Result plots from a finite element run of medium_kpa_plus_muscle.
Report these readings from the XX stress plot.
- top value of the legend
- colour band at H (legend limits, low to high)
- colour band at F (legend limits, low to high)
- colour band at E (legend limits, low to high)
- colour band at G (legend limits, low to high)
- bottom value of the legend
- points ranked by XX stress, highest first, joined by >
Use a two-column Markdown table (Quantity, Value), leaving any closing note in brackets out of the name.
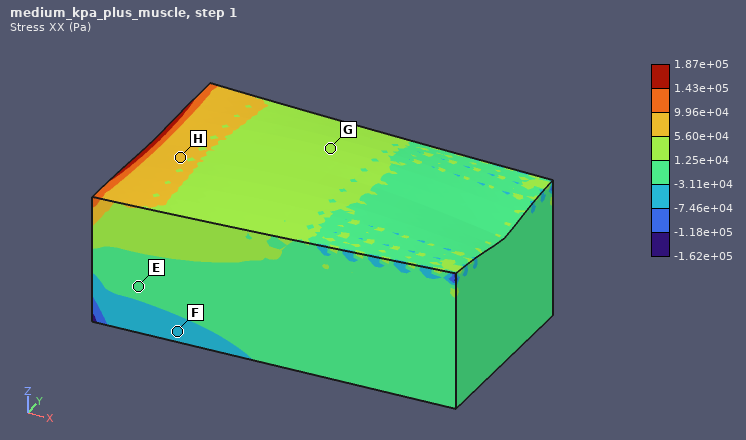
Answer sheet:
| Quantity | Value |
|---|---|
| top value of the legend | 1.87e+05 Pa |
| colour band at H | 5.60e+04 to 9.96e+04 Pa |
| colour band at F | -7.46e+04 to -3.11e+04 Pa |
| colour band at E | -3.11e+04 to 1.25e+04 Pa |
| colour band at G | 1.25e+04 to 5.60e+04 Pa |
| bottom value of the legend | -1.62e+05 Pa |
| points ranked by XX stress, highest first, joined by > | H > G > E > F |
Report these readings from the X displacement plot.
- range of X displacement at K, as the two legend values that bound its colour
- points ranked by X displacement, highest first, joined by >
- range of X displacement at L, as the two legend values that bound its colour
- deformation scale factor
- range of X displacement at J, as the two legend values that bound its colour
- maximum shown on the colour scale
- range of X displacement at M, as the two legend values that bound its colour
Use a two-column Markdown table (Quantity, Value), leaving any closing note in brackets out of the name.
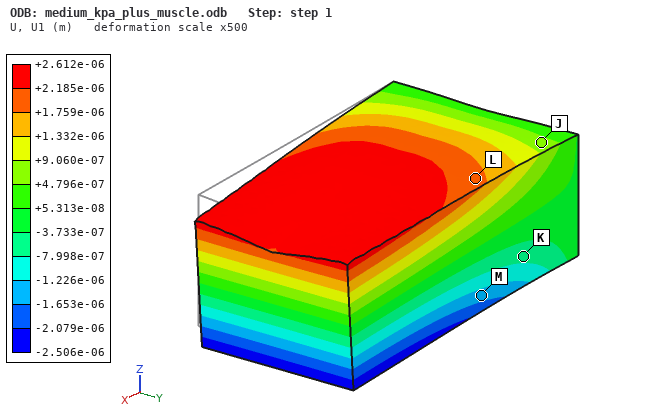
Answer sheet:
| Quantity | Value |
|---|---|
| range of X displacement at K, as the two legend values that bound its colour | -7.998e-07 to -3.733e-07 m |
| points ranked by X displacement, highest first, joined by > | L > J > K > M |
| range of X displacement at L, as the two legend values that bound its colour | +1.759e-06 to +2.185e-06 m |
| deformation scale factor | 500 |
| range of X displacement at J, as the two legend values that bound its colour | +4.796e-07 to +9.060e-07 m |
| maximum shown on the colour scale | +2.612e-06 m |
| range of X displacement at M, as the two legend values that bound its colour | -1.653e-06 to -1.226e-06 m |
